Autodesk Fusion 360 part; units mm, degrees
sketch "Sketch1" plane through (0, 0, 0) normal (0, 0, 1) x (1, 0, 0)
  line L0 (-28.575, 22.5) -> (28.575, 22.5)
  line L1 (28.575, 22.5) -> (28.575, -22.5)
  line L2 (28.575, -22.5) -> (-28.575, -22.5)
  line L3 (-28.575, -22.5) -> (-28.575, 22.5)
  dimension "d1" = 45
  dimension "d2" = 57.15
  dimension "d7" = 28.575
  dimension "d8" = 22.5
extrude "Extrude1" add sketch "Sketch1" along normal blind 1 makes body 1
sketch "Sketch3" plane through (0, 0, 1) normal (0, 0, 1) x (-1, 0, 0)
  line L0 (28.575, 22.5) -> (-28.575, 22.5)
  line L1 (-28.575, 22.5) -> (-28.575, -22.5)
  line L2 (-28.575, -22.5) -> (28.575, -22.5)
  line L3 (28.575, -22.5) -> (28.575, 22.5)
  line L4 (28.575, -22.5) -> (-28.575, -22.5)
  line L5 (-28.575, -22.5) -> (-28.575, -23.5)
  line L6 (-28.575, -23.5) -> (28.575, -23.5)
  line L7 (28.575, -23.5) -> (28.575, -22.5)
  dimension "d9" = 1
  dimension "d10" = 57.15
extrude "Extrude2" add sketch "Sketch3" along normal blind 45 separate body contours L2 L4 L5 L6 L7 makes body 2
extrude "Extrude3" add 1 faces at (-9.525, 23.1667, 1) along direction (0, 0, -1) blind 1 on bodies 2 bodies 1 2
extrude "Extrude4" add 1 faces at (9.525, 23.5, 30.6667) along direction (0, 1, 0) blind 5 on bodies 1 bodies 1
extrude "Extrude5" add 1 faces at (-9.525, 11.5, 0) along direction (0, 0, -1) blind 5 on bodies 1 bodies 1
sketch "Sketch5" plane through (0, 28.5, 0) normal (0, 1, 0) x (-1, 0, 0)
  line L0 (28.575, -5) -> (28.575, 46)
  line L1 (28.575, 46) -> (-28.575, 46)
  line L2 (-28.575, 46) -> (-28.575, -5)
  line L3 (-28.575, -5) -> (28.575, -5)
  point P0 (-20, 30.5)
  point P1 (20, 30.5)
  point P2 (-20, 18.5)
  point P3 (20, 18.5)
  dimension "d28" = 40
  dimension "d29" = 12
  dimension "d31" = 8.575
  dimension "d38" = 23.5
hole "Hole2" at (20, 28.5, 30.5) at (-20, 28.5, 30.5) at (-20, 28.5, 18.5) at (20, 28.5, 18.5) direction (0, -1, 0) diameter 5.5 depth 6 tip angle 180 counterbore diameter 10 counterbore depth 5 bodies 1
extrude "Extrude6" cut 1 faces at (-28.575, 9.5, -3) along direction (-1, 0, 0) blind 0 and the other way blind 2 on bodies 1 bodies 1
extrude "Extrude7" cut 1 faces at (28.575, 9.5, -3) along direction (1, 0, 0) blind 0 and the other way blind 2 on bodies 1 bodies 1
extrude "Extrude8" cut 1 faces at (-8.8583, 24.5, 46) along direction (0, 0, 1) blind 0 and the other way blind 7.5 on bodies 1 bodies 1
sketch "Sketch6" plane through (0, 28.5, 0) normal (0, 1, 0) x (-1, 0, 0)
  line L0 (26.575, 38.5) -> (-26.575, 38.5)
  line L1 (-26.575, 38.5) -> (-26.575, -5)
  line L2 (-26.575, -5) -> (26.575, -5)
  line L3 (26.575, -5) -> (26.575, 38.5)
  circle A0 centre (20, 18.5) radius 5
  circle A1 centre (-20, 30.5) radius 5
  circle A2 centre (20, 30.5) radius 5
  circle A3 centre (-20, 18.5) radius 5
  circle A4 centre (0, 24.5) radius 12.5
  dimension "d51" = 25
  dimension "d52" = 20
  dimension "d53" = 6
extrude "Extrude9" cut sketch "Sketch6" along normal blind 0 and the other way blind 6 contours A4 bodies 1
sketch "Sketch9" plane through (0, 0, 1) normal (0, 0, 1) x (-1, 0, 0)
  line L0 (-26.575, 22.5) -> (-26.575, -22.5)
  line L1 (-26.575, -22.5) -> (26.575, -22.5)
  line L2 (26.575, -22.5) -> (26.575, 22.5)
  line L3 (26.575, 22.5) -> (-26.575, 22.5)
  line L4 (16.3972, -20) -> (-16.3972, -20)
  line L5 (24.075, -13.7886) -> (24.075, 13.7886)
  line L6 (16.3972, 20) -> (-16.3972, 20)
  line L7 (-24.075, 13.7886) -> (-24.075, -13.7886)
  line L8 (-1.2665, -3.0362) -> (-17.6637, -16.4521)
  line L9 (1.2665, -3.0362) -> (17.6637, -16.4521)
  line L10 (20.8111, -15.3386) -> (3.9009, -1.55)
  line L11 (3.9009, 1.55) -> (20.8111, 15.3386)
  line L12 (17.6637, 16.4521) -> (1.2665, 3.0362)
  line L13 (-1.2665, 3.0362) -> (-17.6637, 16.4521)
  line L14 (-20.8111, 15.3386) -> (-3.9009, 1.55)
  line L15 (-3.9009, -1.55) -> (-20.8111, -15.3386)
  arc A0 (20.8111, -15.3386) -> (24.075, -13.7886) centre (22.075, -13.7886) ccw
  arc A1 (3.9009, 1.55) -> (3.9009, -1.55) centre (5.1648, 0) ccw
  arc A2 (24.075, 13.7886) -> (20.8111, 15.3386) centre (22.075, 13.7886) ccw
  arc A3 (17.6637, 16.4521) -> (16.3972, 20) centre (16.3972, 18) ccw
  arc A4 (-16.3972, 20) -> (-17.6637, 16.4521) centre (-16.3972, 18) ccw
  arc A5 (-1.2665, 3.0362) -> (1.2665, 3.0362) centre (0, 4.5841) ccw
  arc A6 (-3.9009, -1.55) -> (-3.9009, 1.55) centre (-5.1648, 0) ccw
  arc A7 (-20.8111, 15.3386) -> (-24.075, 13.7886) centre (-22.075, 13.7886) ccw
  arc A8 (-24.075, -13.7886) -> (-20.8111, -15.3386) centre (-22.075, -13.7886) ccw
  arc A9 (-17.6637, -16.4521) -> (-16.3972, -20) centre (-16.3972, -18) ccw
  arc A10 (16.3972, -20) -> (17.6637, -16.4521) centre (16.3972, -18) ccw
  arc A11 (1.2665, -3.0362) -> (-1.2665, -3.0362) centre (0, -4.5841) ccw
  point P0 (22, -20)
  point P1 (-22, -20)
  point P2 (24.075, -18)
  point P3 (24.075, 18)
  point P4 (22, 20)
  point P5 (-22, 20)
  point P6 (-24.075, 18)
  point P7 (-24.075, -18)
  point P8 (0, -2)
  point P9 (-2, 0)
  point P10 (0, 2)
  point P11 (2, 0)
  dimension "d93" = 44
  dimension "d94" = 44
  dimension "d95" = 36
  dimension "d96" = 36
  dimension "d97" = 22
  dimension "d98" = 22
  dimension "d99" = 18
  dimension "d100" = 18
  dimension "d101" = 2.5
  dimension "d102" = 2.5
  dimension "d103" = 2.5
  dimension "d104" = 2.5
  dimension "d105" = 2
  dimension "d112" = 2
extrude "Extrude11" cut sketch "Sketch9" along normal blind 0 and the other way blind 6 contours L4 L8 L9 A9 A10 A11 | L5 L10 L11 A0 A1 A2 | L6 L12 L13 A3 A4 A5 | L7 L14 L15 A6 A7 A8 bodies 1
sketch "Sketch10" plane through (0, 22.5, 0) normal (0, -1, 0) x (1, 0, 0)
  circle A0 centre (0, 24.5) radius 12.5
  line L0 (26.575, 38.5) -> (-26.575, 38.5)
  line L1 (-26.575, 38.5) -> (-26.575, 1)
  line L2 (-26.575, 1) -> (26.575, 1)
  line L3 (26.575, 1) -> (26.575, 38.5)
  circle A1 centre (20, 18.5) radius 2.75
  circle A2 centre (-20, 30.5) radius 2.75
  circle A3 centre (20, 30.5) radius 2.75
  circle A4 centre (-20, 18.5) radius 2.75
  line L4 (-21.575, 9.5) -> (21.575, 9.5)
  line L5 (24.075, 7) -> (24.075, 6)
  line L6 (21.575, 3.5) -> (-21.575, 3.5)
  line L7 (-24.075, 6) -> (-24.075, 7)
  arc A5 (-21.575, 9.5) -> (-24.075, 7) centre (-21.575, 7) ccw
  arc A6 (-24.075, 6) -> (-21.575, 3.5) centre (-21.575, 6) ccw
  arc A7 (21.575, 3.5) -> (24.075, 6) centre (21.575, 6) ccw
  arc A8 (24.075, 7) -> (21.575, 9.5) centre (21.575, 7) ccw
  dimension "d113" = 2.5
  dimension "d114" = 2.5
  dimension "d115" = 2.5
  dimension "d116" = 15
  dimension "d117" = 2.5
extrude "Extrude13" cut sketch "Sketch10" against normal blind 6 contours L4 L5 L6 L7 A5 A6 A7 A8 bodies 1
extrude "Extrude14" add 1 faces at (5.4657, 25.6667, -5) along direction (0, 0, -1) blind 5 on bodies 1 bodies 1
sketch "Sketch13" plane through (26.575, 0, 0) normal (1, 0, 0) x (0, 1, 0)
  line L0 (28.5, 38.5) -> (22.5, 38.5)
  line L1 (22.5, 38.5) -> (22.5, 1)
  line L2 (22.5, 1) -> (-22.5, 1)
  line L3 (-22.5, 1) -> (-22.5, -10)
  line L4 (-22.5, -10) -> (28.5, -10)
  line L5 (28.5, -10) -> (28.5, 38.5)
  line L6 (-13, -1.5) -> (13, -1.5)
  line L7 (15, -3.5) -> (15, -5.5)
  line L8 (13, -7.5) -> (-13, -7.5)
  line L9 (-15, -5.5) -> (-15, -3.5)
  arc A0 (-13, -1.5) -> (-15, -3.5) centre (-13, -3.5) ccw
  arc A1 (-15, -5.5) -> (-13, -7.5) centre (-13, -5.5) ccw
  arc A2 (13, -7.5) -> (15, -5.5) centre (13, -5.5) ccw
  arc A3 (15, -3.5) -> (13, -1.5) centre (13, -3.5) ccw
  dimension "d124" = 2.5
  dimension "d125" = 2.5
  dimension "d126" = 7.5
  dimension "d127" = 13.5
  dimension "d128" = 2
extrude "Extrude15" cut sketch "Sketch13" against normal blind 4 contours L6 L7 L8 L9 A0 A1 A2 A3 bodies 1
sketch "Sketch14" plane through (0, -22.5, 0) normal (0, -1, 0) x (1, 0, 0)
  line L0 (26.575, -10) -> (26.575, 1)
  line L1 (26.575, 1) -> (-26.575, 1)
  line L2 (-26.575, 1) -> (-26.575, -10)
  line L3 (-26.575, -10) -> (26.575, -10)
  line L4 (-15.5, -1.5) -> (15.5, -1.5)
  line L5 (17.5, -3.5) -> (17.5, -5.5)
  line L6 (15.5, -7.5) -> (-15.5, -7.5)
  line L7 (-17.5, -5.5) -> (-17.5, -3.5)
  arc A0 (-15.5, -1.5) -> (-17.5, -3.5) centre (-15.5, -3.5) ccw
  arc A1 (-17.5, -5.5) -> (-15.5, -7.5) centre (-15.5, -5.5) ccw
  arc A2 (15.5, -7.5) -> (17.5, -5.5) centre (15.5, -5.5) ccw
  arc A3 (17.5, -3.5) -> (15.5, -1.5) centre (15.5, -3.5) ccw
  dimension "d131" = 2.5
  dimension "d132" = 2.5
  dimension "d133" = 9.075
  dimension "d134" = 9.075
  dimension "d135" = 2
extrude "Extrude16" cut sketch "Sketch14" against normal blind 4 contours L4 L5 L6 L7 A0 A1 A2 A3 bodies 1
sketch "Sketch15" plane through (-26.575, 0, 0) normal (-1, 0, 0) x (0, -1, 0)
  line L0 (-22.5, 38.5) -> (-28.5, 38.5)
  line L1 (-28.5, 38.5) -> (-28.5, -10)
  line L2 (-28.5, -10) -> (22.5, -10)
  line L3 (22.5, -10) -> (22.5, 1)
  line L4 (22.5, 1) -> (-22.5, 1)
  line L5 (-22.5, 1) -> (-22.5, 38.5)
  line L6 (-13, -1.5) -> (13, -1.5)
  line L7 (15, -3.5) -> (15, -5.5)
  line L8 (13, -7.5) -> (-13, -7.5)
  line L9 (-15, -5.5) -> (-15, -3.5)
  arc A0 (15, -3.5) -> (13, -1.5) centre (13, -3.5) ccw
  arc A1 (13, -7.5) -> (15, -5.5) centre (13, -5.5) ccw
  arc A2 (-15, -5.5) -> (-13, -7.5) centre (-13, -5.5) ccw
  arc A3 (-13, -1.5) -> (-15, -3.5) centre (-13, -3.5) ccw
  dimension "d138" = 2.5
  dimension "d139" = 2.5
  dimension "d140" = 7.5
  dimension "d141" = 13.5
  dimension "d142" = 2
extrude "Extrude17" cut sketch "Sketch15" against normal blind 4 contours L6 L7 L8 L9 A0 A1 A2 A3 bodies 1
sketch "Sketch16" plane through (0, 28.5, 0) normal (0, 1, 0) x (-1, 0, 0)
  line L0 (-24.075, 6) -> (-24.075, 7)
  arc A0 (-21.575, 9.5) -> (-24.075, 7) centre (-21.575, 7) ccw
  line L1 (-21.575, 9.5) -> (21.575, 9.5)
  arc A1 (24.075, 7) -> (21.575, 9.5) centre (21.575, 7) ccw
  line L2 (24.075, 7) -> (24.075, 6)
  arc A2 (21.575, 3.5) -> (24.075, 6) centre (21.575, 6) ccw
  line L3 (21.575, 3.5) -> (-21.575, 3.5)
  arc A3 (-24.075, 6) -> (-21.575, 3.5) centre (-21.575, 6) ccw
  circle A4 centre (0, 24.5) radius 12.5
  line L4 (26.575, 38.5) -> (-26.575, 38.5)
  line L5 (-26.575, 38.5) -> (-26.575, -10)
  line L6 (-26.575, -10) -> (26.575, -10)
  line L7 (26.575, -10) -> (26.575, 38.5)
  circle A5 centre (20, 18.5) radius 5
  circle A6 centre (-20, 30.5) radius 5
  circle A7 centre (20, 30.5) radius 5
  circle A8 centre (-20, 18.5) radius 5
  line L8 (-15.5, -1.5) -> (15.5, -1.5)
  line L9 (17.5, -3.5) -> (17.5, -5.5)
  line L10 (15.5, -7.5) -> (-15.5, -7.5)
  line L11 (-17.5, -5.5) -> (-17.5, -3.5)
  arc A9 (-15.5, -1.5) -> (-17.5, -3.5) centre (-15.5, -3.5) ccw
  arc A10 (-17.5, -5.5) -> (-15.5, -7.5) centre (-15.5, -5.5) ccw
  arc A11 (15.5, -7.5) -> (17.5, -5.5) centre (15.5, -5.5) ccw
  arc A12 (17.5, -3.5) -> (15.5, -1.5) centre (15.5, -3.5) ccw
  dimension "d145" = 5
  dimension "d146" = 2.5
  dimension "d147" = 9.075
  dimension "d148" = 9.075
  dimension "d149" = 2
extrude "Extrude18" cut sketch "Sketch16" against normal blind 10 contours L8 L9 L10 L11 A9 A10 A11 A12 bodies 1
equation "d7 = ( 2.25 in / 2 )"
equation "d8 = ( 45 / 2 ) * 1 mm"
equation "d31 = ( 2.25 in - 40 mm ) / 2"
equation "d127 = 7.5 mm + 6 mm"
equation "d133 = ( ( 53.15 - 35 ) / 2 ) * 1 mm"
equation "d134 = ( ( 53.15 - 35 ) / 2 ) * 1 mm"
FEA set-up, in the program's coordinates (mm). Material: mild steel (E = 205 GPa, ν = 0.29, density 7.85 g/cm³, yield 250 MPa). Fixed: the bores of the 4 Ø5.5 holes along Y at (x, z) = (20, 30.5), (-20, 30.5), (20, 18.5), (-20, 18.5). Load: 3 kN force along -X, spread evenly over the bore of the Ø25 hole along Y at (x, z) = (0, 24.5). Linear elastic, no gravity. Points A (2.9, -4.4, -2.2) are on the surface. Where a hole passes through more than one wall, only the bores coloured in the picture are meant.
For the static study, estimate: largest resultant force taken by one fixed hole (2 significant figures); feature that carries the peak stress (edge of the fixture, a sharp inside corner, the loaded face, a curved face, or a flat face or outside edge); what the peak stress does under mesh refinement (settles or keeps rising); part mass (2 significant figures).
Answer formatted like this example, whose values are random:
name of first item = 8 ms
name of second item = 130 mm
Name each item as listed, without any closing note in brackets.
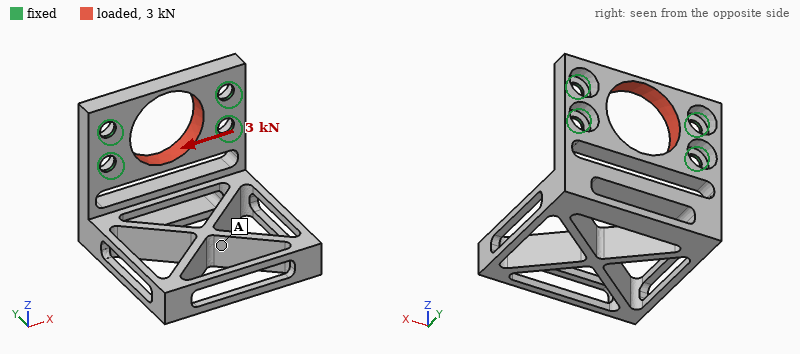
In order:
largest resultant force taken by one fixed hole = 760 N
feature that carries the peak stress = edge of the fixture
what the peak stress does under mesh refinement = keeps rising
part mass = 120 g
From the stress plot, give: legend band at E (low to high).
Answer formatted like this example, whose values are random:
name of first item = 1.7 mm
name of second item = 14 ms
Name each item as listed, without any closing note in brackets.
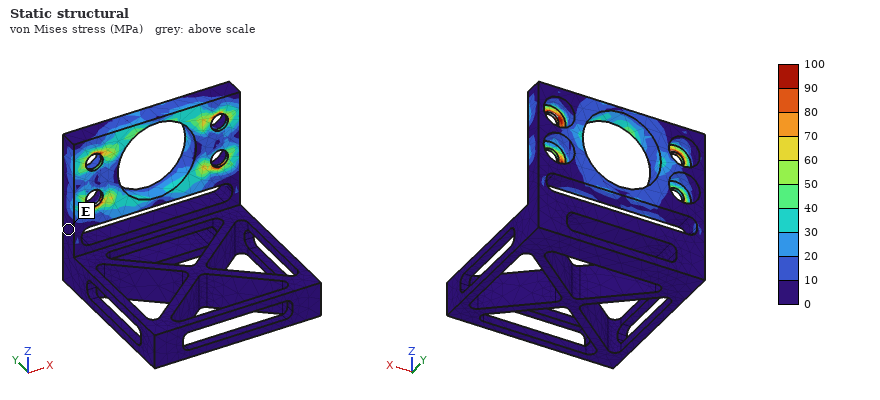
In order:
legend band at E = 0 to 10 MPa
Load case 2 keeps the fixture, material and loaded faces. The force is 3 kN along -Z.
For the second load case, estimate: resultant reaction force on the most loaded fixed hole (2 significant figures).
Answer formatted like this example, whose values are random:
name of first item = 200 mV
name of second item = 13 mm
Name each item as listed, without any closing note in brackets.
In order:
resultant reaction force on the most loaded fixed hole = 830 N
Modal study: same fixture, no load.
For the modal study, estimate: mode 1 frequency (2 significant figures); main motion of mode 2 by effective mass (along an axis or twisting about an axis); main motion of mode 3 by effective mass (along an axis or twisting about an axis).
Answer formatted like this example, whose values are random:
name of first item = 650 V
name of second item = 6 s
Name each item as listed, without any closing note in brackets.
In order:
mode 1 frequency = 670 Hz
main motion of mode 2 by effective mass = along X
main motion of mode 3 by effective mass = along Y
